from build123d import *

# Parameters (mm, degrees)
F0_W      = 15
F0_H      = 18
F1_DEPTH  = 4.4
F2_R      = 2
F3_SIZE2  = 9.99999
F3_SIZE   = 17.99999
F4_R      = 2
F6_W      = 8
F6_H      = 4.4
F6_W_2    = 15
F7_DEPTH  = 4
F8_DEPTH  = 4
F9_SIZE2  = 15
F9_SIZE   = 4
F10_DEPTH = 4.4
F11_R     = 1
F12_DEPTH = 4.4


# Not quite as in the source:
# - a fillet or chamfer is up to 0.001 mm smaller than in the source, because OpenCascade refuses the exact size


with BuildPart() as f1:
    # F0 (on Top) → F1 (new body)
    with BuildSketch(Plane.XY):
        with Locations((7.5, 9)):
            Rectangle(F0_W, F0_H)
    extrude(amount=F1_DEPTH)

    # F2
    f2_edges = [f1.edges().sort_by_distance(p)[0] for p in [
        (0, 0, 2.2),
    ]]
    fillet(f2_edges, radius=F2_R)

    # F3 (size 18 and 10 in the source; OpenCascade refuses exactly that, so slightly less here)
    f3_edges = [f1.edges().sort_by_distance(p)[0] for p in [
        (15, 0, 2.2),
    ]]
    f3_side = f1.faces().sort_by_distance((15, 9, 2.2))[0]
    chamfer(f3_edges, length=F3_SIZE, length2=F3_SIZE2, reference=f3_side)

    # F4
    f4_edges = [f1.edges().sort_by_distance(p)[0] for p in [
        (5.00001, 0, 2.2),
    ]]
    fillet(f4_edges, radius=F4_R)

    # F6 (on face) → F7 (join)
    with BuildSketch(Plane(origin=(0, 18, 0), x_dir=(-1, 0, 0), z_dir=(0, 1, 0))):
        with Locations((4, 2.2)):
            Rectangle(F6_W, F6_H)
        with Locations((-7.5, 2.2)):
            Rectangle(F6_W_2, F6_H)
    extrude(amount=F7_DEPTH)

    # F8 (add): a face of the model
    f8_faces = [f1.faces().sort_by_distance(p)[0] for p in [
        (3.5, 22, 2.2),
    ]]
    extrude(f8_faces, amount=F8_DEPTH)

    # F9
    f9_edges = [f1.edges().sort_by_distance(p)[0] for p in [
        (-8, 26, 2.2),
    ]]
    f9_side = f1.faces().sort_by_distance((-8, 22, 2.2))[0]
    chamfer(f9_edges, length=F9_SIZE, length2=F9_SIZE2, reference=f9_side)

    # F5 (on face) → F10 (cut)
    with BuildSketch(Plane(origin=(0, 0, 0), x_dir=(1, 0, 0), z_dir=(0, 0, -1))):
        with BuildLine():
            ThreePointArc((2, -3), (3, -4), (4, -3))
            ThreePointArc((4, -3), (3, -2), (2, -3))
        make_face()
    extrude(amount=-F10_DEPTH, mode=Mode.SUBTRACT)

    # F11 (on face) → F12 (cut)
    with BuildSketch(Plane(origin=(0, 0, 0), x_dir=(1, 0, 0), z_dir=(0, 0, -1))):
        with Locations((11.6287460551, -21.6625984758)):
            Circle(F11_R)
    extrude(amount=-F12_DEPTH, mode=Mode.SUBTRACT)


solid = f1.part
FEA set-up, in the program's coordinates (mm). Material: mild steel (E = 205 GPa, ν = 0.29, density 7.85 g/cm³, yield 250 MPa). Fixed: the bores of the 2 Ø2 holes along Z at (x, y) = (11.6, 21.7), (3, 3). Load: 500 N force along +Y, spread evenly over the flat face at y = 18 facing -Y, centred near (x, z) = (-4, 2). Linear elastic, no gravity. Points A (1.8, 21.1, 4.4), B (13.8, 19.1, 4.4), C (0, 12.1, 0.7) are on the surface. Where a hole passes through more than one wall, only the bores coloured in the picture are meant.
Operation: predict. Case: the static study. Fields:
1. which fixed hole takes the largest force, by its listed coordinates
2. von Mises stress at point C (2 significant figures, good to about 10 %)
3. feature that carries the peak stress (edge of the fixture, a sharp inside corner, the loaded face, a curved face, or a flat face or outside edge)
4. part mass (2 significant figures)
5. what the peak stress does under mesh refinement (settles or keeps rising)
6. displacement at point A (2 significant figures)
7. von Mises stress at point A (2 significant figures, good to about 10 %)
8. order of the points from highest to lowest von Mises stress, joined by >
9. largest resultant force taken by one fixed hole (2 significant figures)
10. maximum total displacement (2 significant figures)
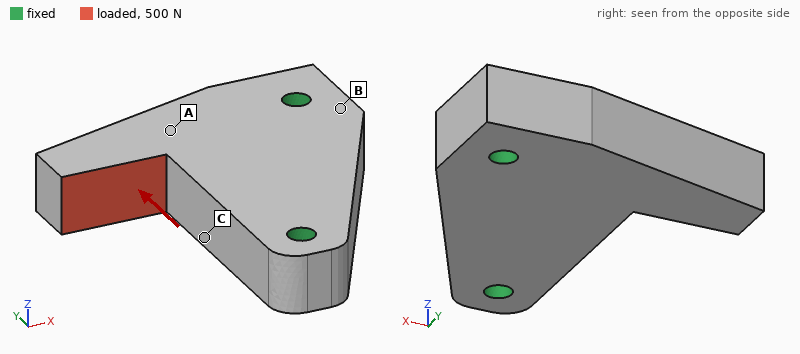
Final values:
(3, 3)
36 MPa
a sharp inside corner
11 g
keeps rising
1.9 µm
19 MPa
C > A > B
490 N
11 µm
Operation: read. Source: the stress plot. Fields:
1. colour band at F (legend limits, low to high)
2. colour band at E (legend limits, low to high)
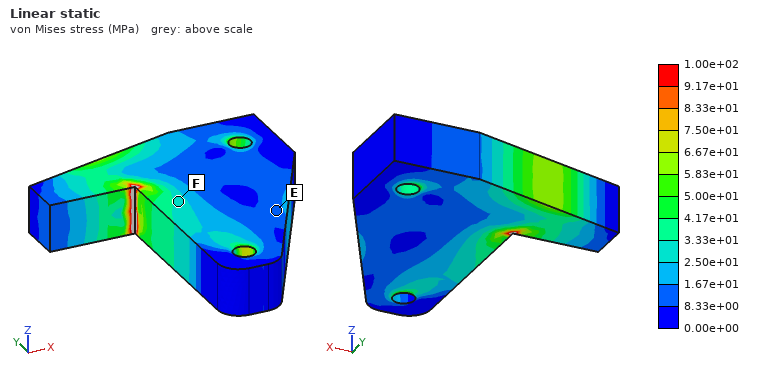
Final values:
2.50e+01 to 3.33e+01 MPa
8.33e+00 to 1.67e+01 MPa
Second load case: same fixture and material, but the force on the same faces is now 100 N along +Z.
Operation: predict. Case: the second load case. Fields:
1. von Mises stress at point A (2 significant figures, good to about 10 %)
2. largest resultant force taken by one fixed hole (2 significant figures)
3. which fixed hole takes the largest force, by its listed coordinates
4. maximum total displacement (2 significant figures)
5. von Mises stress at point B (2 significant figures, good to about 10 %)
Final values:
25 MPa
57 N
(11.6, 21.7)
11 µm
9.8 MPa
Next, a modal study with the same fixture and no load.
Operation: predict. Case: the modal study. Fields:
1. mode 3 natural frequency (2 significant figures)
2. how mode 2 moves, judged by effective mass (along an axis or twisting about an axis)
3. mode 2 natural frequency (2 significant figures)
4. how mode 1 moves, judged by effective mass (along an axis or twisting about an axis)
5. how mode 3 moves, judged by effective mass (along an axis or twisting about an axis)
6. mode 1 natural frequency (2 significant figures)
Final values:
40 kHz
along Y
32 kHz
along Z
along Z
14 kHz
